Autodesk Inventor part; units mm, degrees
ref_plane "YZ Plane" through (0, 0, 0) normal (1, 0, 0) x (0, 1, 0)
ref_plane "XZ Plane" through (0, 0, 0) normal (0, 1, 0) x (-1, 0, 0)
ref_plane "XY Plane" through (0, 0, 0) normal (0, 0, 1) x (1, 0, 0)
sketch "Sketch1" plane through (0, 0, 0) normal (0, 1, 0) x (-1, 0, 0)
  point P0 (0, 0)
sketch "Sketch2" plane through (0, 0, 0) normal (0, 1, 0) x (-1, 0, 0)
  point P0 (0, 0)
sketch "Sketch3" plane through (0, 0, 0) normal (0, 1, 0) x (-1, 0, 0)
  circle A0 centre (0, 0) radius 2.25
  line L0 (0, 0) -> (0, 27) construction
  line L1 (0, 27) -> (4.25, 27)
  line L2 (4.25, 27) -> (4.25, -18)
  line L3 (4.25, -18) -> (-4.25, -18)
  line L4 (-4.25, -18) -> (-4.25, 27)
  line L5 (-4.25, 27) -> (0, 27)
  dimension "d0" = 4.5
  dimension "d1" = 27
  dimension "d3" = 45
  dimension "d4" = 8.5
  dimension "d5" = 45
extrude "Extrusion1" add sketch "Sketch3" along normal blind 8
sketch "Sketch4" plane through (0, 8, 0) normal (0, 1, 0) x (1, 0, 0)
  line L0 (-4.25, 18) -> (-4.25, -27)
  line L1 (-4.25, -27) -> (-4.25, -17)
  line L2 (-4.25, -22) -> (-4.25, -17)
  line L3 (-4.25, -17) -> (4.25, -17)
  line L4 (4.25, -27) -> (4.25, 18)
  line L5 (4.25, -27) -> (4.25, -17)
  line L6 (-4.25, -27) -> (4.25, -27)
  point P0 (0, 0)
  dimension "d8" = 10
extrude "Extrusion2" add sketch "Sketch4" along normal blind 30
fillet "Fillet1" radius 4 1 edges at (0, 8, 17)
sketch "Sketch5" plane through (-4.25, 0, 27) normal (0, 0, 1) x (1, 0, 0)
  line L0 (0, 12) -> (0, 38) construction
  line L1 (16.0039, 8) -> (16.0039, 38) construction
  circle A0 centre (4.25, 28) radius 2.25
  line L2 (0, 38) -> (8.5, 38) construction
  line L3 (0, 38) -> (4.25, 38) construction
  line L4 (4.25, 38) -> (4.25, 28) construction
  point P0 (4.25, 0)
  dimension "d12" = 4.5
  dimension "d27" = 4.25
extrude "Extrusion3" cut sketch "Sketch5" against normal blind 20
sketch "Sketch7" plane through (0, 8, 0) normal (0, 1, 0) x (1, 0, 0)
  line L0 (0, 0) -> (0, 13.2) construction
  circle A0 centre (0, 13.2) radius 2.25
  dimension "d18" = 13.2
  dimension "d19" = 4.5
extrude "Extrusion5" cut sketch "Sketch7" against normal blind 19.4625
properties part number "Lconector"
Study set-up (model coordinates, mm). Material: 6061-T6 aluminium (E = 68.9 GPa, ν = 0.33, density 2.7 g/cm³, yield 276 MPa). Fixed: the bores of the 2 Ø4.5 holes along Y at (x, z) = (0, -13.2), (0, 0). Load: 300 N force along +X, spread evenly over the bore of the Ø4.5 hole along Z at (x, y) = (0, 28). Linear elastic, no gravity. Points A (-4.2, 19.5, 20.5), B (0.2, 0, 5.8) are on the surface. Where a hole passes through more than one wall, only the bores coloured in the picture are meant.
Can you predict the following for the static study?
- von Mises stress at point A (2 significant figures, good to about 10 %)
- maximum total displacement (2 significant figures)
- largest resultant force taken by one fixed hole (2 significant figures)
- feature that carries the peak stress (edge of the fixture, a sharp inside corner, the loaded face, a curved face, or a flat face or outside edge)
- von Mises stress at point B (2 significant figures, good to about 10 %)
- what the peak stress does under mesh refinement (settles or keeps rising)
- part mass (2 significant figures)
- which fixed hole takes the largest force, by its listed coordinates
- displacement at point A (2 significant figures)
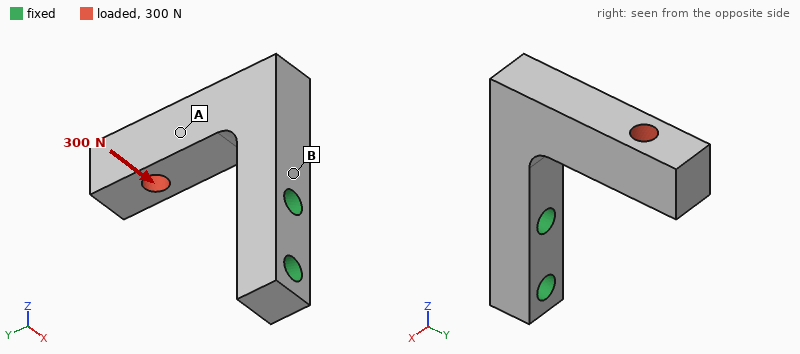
22 MPa
0.34 mm
380 N
edge of the fixture
88 MPa
keeps rising
14 g
(0, 0)
0.16 mm
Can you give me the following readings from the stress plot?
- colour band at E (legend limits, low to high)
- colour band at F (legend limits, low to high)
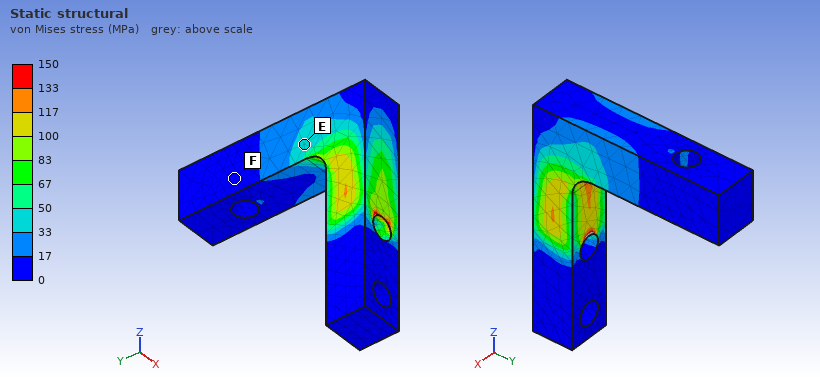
33 to 50 MPa
0 to 17 MPa
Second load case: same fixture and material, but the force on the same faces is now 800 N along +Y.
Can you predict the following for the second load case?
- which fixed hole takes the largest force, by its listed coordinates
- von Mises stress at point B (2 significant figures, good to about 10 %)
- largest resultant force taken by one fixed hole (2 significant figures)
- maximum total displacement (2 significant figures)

(0, 0)
160 MPa
850 N
0.27 mm
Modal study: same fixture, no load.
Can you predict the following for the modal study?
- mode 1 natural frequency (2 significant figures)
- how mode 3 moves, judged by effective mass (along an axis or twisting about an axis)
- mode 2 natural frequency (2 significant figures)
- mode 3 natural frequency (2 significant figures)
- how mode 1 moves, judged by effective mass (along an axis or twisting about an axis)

2500 Hz
along X
2800 Hz
7200 Hz
along X
